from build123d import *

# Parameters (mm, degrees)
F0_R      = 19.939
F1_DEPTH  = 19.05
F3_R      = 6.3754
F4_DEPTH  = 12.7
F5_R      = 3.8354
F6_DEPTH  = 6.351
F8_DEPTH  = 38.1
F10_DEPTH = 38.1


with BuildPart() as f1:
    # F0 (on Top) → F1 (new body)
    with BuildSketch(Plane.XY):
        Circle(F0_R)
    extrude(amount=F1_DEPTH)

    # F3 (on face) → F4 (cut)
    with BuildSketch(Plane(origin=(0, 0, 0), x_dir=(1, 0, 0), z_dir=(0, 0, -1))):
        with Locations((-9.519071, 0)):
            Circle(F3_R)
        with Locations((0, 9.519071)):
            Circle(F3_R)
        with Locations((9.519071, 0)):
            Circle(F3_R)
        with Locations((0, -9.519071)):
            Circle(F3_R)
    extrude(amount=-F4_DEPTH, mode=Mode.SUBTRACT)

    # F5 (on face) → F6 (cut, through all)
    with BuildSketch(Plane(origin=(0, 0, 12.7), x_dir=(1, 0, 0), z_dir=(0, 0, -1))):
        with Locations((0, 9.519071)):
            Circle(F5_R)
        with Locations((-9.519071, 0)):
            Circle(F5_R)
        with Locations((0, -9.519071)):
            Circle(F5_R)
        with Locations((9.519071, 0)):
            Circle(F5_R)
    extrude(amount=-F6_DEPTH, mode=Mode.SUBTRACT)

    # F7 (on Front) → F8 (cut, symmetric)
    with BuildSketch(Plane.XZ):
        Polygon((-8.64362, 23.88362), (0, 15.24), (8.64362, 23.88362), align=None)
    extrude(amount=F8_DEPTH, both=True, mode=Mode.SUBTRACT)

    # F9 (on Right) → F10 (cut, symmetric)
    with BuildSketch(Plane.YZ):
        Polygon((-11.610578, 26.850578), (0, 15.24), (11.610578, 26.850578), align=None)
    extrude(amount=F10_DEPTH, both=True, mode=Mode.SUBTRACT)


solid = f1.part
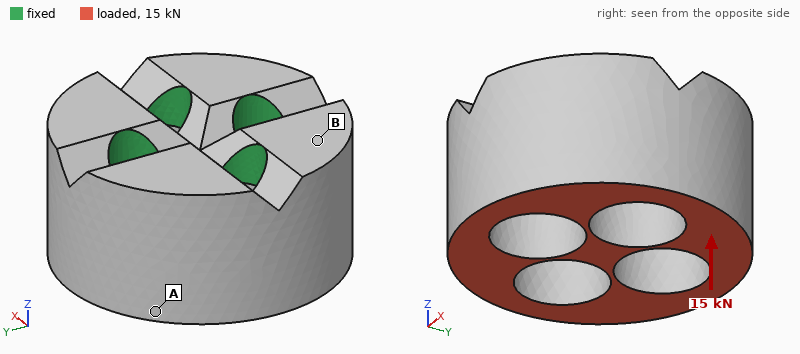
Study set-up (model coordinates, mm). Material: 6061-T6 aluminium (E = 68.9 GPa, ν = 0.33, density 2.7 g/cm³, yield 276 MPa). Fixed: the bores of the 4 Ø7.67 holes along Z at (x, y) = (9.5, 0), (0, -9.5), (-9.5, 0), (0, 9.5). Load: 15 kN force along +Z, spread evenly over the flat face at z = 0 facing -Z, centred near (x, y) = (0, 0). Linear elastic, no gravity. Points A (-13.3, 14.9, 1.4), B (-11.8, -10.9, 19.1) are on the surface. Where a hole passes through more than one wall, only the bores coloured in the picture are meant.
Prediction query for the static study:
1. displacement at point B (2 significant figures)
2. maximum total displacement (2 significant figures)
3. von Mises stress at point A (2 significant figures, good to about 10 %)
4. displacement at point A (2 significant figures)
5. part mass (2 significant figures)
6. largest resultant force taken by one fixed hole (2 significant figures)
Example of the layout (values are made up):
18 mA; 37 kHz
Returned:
8.5 µm; 15 µm; 28 MPa; 14 µm; 42 g; 3.8 kN
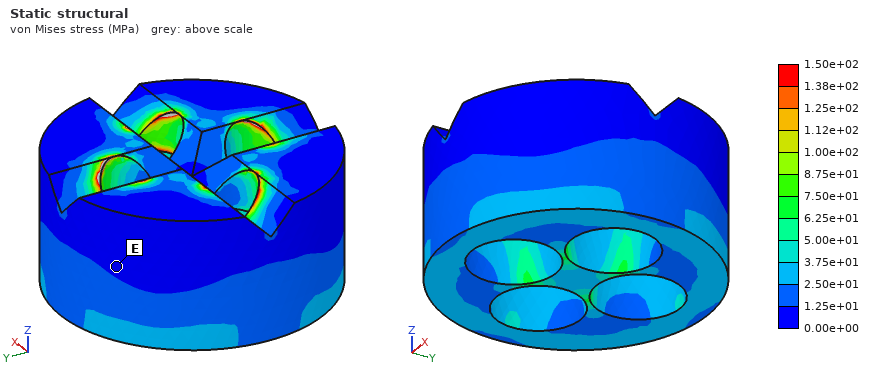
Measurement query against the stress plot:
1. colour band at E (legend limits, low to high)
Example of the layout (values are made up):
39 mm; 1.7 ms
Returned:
0.00e+00 to 1.25e+01 MPa
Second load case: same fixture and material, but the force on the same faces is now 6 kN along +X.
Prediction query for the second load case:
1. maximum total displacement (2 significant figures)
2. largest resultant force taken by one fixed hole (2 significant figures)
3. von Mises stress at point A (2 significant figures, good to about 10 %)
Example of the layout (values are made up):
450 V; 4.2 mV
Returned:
30 µm; 3.0 kN; 16 MPa
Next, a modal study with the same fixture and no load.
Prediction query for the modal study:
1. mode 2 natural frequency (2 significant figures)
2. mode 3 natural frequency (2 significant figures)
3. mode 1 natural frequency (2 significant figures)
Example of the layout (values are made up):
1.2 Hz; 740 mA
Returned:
20 kHz; 23 kHz; 20 kHz
